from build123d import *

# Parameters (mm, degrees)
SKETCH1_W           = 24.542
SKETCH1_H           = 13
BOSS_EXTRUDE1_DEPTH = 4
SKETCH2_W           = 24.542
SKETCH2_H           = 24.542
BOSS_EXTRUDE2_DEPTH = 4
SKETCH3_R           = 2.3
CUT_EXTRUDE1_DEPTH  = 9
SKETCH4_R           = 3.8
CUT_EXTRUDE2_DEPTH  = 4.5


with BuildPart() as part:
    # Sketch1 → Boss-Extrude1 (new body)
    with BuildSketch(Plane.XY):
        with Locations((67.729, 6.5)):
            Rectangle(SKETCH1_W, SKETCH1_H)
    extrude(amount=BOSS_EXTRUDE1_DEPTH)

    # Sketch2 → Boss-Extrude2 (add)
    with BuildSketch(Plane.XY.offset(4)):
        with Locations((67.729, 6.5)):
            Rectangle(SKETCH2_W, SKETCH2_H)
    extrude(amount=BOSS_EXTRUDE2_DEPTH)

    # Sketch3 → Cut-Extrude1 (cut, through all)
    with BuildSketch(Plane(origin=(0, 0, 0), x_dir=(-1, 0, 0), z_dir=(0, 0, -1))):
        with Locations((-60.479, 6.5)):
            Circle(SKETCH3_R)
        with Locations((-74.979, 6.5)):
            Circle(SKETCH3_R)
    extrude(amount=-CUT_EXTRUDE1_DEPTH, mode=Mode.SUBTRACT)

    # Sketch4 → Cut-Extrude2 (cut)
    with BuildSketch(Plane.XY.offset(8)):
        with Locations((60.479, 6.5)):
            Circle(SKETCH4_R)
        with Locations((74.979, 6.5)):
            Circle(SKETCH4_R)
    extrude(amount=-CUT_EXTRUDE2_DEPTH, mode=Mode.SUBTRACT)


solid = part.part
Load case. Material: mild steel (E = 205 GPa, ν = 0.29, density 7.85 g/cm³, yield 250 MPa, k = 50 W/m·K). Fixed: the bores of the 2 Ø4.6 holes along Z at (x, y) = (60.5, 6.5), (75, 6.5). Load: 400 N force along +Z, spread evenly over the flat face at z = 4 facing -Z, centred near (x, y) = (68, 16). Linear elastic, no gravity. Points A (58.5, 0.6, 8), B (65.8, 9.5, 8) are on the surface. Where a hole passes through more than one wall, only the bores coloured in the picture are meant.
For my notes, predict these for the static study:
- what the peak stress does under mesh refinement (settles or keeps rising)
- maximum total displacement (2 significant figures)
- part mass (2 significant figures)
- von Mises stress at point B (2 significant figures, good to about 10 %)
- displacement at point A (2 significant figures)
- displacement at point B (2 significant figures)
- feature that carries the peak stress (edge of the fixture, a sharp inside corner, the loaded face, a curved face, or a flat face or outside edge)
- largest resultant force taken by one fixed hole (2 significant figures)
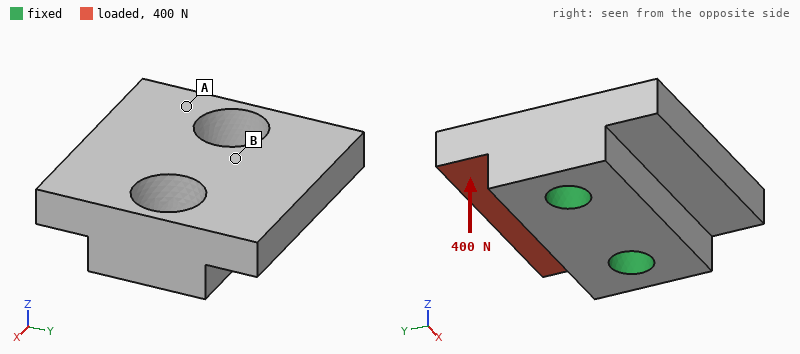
keeps rising
4.3 µm
25 g
17 MPa
1.1 µm
1.4 µm
edge of the fixture
200 N
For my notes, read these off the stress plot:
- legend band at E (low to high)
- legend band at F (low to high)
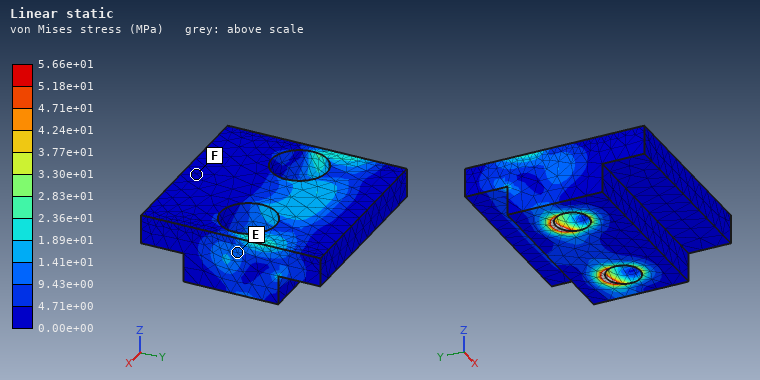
9.43e+00 to 1.41e+01 MPa
0.00e+00 to 4.71e+00 MPa
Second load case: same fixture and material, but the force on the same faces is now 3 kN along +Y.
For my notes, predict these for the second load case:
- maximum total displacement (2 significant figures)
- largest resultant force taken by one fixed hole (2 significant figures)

4.5 µm
1.5 kN
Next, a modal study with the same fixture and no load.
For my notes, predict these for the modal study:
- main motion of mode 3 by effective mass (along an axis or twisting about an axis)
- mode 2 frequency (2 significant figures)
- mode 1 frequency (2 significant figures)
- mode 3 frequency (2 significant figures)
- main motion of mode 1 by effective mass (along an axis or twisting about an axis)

along Z
32 kHz
19 kHz
34 kHz
along Y
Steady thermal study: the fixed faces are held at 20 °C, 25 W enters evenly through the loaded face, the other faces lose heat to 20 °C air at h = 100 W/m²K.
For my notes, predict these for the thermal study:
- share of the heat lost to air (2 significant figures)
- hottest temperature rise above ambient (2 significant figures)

10.0 %
48 K
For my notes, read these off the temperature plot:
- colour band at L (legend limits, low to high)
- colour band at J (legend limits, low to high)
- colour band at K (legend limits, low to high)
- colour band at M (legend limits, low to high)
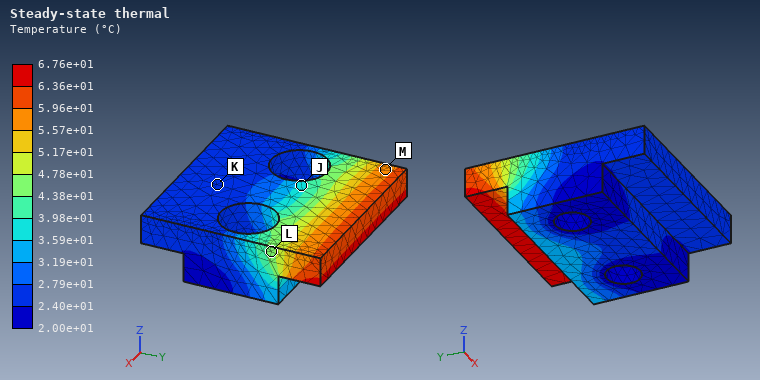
4.38e+01 to 4.78e+01 °C
3.59e+01 to 3.98e+01 °C
2.40e+01 to 2.79e+01 °C
5.57e+01 to 5.96e+01 °C
